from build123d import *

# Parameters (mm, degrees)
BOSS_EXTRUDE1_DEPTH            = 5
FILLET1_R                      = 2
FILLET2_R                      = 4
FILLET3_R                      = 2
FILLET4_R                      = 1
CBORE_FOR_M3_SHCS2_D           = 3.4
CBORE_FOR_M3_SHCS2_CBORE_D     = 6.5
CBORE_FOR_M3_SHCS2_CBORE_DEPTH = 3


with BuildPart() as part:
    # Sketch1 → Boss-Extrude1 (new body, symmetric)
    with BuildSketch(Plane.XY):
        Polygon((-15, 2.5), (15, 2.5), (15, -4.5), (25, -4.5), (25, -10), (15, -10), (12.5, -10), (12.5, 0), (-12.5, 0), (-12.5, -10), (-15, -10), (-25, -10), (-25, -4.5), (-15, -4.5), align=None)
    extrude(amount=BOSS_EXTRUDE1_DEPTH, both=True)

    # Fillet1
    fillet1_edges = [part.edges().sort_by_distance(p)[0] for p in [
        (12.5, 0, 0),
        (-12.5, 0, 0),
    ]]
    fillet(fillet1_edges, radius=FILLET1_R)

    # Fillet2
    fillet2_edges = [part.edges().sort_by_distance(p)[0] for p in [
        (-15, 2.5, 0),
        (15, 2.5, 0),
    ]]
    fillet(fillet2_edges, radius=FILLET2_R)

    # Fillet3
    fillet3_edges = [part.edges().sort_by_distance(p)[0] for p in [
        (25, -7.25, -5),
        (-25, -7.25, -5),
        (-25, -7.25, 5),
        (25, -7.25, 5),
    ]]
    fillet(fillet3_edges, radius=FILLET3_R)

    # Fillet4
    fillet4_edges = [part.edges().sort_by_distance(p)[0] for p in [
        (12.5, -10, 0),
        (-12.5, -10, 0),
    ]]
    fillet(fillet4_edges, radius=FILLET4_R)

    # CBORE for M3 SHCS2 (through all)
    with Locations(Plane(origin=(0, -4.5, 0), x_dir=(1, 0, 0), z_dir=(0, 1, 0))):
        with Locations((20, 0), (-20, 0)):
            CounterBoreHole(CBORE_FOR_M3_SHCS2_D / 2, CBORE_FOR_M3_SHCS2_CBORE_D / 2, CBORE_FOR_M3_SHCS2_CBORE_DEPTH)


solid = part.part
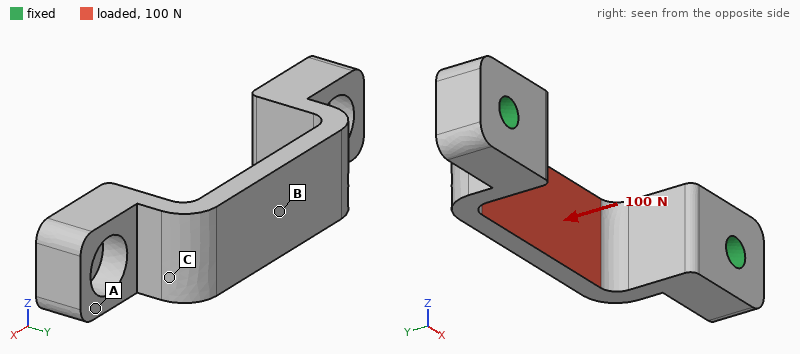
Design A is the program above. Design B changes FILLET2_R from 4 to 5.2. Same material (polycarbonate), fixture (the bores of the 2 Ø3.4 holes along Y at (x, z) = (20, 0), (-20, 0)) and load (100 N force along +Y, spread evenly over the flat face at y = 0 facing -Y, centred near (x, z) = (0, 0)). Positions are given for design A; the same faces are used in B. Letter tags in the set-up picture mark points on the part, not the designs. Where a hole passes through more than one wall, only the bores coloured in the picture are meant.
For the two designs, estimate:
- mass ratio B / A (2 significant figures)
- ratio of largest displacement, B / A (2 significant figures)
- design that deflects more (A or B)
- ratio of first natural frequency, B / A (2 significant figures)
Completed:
0.98
1.1
B
1.0
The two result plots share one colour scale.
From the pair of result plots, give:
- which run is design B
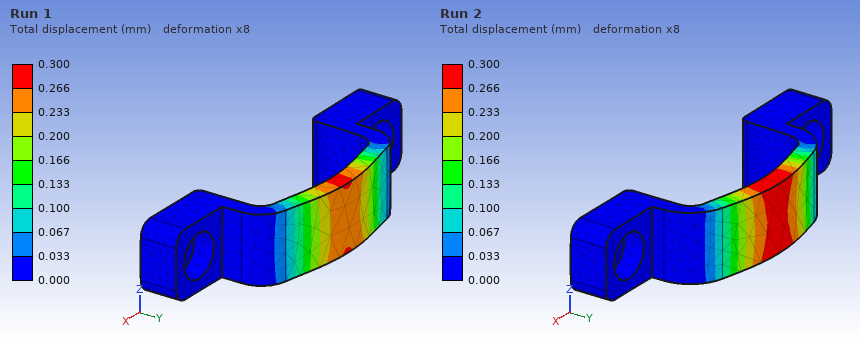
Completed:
Run 2
